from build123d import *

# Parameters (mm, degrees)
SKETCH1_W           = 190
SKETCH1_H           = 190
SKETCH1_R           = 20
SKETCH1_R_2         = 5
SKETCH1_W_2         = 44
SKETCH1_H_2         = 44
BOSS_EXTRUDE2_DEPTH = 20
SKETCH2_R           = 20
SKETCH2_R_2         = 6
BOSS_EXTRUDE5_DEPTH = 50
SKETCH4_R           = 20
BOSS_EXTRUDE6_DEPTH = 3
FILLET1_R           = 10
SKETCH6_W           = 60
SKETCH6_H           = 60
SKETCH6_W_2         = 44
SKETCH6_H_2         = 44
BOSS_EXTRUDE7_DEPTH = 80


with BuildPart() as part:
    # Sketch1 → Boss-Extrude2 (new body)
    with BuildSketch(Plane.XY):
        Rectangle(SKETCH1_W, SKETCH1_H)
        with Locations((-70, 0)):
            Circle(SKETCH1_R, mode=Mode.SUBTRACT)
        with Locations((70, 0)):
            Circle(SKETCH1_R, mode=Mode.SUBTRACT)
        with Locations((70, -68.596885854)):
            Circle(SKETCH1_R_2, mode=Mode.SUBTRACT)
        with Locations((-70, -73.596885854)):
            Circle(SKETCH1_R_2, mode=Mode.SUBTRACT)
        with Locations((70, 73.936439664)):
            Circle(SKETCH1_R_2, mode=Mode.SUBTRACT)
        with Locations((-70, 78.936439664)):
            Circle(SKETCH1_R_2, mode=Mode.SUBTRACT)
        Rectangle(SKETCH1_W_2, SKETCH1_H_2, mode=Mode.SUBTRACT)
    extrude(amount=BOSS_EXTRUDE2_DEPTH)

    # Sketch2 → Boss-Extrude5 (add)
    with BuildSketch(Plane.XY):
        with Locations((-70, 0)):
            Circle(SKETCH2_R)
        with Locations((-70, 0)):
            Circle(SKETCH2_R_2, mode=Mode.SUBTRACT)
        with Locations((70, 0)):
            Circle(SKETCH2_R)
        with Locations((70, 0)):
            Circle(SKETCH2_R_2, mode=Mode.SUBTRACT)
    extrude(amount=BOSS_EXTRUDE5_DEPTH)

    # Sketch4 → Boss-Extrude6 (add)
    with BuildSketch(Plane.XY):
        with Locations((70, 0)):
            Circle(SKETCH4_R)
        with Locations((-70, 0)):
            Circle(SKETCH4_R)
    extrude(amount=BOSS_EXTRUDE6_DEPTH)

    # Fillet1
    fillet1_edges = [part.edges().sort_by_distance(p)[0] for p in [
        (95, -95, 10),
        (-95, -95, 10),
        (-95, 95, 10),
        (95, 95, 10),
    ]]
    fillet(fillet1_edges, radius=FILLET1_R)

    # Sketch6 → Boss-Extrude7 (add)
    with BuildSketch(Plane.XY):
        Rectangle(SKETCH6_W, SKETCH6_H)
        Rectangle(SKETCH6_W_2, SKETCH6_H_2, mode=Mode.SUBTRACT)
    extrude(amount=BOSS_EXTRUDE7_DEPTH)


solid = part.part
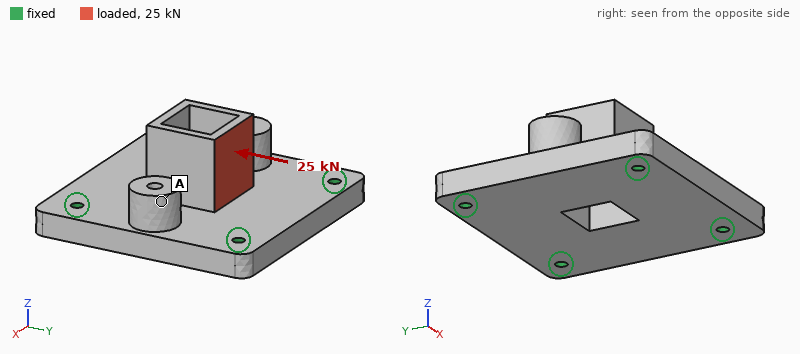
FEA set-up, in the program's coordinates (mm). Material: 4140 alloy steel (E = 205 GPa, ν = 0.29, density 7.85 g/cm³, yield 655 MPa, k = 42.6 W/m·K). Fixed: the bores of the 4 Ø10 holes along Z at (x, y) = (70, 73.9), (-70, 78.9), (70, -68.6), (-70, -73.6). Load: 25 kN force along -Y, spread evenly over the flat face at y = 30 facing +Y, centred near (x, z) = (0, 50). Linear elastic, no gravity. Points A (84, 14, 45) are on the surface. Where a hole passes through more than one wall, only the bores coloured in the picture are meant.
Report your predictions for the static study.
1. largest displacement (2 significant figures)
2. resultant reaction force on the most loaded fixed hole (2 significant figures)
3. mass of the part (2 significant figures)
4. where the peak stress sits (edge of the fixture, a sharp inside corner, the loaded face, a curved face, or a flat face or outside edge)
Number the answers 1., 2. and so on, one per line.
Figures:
1. 84 µm
2. 8.0 kN
3. 6.6 kg
4. the loaded face
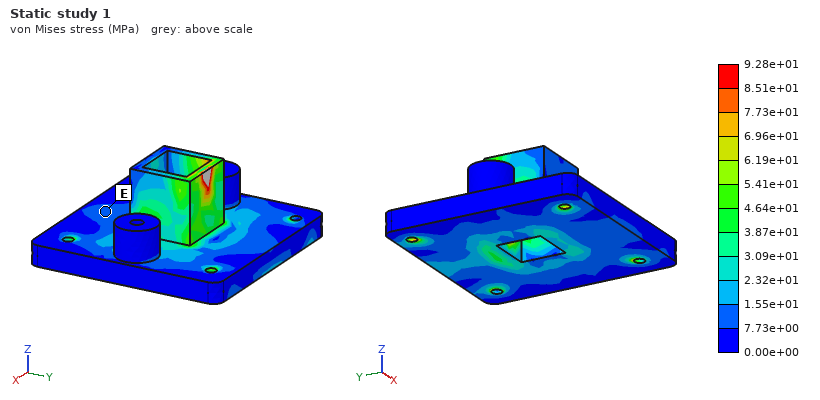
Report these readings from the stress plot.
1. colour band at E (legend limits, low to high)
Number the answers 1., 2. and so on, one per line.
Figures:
1. 7.73e+00 to 1.55e+01 MPa
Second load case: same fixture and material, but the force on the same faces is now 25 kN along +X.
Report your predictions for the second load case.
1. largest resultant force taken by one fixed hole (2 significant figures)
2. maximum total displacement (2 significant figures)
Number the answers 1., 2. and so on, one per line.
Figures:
1. 11 kN
2. 77 µm
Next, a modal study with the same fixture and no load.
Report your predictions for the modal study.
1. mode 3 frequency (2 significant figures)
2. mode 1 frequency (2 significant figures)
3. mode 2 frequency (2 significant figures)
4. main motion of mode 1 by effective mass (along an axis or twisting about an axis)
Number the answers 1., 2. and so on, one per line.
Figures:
1. 3700 Hz
2. 2600 Hz
3. 3400 Hz
4. along Z
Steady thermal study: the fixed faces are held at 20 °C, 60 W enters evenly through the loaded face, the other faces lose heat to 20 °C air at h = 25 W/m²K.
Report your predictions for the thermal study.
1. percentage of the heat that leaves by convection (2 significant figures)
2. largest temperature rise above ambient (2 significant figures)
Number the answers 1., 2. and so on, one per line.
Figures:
1. 45 %
2. 56 K
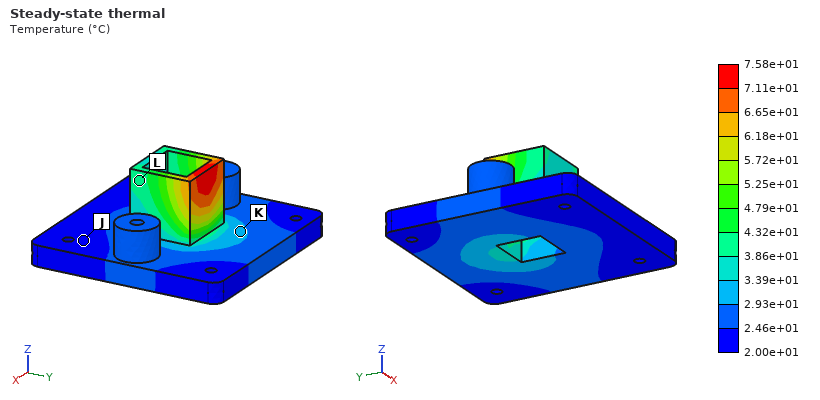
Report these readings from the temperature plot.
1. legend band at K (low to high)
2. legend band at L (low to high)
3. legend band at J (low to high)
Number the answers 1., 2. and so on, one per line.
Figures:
1. 2.93e+01 to 3.39e+01 °C
2. 3.86e+01 to 4.32e+01 °C
3. 2.00e+01 to 2.46e+01 °C
